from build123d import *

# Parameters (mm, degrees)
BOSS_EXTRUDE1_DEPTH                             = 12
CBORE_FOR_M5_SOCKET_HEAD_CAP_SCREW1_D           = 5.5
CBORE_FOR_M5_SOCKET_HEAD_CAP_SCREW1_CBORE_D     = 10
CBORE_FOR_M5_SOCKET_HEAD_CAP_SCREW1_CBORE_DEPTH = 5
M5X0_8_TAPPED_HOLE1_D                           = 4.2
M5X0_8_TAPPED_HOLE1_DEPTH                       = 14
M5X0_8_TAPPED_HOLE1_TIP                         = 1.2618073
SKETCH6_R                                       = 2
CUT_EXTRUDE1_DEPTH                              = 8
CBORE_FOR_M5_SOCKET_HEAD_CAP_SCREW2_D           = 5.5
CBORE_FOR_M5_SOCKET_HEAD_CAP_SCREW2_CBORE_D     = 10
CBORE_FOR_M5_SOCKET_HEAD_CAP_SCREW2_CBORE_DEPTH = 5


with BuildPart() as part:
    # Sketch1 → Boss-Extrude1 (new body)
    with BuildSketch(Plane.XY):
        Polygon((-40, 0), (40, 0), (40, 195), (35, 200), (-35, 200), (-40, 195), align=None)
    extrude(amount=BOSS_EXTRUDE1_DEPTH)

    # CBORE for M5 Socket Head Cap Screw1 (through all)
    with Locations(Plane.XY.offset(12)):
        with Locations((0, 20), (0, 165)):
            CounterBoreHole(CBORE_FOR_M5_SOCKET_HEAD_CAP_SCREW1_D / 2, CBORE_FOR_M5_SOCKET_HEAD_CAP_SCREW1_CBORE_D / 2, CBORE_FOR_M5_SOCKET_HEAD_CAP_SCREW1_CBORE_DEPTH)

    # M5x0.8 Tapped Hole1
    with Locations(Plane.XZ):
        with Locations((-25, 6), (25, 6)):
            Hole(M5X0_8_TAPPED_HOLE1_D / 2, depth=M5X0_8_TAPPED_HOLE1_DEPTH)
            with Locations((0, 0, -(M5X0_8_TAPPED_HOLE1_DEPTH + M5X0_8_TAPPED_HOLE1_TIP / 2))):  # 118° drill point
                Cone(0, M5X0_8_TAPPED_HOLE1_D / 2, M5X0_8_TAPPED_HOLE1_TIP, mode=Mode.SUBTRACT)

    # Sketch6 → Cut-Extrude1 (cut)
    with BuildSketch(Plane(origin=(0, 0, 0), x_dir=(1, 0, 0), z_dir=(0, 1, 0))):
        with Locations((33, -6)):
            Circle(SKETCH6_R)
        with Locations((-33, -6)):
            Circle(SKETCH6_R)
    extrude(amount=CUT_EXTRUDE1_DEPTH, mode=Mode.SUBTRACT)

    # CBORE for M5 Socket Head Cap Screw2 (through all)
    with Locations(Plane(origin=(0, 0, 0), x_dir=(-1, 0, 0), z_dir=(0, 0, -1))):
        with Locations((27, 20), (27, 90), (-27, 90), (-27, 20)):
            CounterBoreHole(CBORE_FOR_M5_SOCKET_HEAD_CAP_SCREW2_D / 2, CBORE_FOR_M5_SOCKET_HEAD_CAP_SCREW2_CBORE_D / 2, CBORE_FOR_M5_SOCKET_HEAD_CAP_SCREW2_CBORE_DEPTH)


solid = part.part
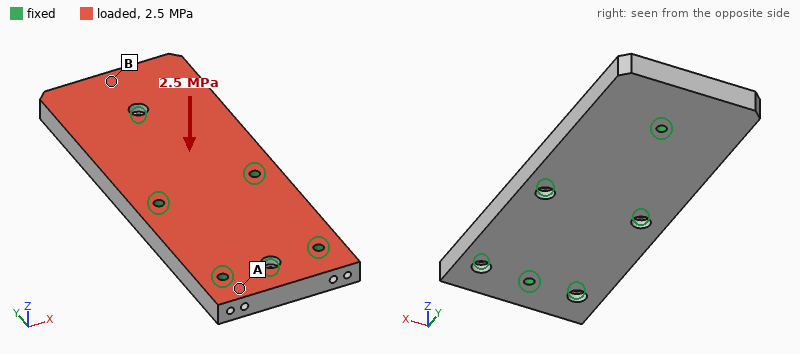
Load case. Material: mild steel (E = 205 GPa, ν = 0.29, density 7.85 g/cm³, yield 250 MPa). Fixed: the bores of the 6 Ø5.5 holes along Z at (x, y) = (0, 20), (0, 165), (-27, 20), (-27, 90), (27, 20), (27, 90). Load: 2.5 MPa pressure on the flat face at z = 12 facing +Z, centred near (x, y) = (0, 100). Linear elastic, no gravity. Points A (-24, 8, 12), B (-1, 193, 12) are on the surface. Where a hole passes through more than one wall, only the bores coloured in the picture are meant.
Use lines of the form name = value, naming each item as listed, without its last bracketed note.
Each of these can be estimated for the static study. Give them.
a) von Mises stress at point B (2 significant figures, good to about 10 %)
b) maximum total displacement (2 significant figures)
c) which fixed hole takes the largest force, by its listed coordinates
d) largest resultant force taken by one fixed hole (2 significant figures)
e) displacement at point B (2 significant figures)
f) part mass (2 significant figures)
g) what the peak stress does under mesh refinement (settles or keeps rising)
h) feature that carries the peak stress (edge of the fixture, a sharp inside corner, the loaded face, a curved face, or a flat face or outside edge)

von Mises stress at point B = 52 MPa
maximum total displacement = 49 µm
which fixed hole takes the largest force, by its listed coordinates = (0, 165)
largest resultant force taken by one fixed hole = 14 kN
displacement at point B = 28 µm
part mass = 1.5 kg
what the peak stress does under mesh refinement = keeps rising
feature that carries the peak stress = edge of the fixture
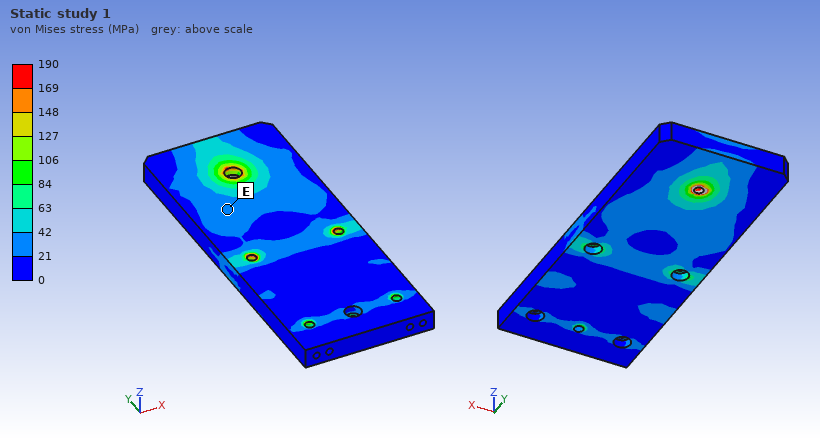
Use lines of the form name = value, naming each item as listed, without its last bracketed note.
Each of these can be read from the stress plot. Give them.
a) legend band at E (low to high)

legend band at E = 21 to 42 MPa
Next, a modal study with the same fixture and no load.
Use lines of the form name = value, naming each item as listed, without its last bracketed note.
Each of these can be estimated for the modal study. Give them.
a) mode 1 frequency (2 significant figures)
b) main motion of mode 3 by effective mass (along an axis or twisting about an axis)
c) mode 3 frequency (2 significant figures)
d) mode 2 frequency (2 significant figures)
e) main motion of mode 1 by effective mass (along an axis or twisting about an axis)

mode 1 frequency = 3000 Hz
main motion of mode 3 by effective mass = along Z
mode 3 frequency = 5600 Hz
mode 2 frequency = 4200 Hz
main motion of mode 1 by effective mass = twisting about Y
